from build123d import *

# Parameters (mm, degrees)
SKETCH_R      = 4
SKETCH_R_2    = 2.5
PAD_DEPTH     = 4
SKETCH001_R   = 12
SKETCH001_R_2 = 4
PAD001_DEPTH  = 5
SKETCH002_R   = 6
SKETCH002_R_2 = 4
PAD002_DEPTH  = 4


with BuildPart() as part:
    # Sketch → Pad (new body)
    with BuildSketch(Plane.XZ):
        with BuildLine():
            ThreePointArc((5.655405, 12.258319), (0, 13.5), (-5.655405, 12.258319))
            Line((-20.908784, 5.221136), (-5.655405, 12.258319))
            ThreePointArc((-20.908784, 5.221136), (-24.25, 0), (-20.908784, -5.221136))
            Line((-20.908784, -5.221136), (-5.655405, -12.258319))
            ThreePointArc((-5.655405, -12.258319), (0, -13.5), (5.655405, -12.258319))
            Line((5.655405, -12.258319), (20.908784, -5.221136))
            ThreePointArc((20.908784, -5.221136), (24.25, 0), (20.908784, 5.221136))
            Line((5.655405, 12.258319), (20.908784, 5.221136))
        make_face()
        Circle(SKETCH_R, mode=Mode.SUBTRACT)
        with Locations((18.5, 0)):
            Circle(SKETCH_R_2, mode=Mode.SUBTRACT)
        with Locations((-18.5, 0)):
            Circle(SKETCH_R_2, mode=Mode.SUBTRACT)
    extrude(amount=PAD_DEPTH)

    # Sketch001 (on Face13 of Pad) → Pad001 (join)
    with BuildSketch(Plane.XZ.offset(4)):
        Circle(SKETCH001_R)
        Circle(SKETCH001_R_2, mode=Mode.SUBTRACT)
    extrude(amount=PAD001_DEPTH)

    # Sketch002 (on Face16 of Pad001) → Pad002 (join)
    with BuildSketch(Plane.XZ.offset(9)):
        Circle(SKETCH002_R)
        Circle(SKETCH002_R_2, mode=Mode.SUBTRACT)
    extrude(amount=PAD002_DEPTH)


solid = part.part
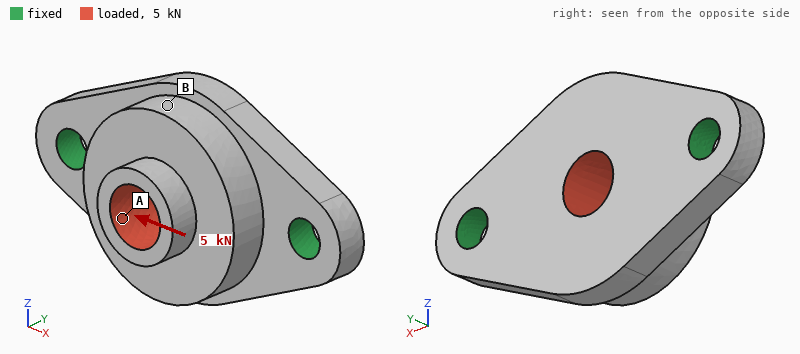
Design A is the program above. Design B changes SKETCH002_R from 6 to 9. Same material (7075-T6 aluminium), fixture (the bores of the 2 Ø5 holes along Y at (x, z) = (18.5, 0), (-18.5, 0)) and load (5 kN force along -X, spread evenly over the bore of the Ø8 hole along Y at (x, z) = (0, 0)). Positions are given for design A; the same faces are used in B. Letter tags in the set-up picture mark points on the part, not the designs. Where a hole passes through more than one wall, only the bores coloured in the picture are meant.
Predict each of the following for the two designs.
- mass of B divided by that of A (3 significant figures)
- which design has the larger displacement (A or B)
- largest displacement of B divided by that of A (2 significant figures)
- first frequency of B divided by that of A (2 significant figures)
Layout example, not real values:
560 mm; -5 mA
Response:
1.10; A; 0.76; 0.90
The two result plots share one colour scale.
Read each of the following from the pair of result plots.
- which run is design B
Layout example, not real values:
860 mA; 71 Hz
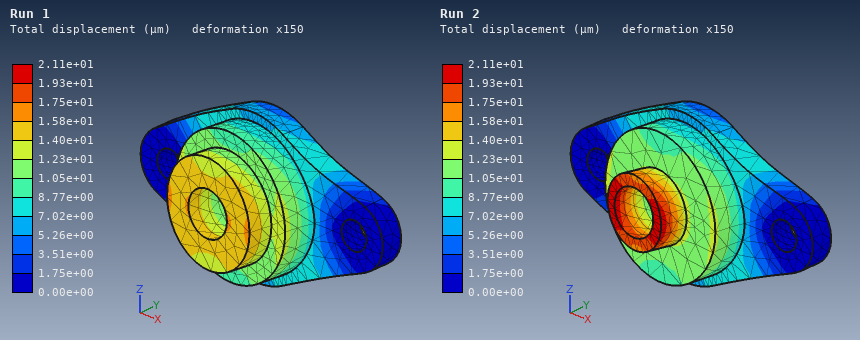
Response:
Run 1
